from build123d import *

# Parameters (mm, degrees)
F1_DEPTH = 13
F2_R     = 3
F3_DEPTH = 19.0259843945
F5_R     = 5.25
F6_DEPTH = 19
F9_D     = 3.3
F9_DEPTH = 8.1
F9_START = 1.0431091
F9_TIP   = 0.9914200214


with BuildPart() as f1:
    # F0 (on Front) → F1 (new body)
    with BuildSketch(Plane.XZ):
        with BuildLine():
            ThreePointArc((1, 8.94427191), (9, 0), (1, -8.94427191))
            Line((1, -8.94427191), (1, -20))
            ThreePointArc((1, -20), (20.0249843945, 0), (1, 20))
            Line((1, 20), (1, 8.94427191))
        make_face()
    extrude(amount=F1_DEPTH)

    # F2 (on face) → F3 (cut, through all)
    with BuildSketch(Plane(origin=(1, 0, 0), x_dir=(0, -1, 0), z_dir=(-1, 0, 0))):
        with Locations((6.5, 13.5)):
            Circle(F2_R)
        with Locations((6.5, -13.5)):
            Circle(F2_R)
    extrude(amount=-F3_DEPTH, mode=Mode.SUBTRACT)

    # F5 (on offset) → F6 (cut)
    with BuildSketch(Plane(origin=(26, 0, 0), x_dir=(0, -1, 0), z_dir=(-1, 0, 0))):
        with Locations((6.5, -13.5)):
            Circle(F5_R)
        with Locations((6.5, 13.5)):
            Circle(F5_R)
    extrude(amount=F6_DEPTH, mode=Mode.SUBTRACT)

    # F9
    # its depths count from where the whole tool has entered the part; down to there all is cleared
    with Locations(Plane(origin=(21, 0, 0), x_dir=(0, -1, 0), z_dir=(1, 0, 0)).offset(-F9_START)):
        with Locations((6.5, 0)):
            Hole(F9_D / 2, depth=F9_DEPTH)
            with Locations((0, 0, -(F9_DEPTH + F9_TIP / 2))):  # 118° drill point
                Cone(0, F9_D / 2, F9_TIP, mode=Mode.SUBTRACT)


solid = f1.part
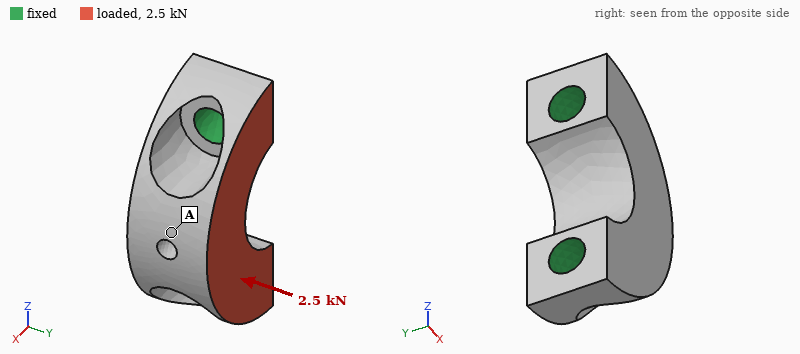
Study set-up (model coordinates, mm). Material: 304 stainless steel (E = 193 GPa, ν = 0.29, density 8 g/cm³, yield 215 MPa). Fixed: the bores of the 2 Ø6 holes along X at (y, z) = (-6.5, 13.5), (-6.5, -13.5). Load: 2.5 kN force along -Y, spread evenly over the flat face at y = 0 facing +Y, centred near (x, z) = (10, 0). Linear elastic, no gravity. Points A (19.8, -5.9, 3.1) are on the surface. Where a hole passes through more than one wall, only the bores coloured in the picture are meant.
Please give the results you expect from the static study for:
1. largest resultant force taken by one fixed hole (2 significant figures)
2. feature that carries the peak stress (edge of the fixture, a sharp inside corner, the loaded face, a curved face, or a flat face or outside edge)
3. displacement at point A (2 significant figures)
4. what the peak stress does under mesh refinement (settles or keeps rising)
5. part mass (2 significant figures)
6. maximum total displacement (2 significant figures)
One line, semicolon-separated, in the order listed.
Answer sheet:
1.3 kN; edge of the fixture; 8.4 µm; keeps rising; 37 g; 9.2 µm
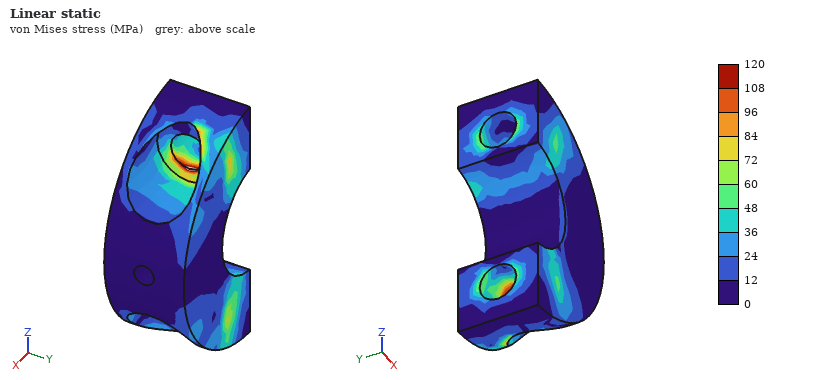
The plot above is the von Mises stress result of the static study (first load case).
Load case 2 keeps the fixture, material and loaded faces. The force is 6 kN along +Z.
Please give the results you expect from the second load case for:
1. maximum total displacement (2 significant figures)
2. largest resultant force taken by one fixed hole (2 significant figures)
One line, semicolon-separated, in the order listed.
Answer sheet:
11 µm; 3.3 kN
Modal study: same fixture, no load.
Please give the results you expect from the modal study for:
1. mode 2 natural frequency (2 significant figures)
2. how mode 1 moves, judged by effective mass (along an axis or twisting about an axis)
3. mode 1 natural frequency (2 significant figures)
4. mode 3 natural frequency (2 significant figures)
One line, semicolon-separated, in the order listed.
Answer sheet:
35 kHz; along Y; 16 kHz; 35 kHz
